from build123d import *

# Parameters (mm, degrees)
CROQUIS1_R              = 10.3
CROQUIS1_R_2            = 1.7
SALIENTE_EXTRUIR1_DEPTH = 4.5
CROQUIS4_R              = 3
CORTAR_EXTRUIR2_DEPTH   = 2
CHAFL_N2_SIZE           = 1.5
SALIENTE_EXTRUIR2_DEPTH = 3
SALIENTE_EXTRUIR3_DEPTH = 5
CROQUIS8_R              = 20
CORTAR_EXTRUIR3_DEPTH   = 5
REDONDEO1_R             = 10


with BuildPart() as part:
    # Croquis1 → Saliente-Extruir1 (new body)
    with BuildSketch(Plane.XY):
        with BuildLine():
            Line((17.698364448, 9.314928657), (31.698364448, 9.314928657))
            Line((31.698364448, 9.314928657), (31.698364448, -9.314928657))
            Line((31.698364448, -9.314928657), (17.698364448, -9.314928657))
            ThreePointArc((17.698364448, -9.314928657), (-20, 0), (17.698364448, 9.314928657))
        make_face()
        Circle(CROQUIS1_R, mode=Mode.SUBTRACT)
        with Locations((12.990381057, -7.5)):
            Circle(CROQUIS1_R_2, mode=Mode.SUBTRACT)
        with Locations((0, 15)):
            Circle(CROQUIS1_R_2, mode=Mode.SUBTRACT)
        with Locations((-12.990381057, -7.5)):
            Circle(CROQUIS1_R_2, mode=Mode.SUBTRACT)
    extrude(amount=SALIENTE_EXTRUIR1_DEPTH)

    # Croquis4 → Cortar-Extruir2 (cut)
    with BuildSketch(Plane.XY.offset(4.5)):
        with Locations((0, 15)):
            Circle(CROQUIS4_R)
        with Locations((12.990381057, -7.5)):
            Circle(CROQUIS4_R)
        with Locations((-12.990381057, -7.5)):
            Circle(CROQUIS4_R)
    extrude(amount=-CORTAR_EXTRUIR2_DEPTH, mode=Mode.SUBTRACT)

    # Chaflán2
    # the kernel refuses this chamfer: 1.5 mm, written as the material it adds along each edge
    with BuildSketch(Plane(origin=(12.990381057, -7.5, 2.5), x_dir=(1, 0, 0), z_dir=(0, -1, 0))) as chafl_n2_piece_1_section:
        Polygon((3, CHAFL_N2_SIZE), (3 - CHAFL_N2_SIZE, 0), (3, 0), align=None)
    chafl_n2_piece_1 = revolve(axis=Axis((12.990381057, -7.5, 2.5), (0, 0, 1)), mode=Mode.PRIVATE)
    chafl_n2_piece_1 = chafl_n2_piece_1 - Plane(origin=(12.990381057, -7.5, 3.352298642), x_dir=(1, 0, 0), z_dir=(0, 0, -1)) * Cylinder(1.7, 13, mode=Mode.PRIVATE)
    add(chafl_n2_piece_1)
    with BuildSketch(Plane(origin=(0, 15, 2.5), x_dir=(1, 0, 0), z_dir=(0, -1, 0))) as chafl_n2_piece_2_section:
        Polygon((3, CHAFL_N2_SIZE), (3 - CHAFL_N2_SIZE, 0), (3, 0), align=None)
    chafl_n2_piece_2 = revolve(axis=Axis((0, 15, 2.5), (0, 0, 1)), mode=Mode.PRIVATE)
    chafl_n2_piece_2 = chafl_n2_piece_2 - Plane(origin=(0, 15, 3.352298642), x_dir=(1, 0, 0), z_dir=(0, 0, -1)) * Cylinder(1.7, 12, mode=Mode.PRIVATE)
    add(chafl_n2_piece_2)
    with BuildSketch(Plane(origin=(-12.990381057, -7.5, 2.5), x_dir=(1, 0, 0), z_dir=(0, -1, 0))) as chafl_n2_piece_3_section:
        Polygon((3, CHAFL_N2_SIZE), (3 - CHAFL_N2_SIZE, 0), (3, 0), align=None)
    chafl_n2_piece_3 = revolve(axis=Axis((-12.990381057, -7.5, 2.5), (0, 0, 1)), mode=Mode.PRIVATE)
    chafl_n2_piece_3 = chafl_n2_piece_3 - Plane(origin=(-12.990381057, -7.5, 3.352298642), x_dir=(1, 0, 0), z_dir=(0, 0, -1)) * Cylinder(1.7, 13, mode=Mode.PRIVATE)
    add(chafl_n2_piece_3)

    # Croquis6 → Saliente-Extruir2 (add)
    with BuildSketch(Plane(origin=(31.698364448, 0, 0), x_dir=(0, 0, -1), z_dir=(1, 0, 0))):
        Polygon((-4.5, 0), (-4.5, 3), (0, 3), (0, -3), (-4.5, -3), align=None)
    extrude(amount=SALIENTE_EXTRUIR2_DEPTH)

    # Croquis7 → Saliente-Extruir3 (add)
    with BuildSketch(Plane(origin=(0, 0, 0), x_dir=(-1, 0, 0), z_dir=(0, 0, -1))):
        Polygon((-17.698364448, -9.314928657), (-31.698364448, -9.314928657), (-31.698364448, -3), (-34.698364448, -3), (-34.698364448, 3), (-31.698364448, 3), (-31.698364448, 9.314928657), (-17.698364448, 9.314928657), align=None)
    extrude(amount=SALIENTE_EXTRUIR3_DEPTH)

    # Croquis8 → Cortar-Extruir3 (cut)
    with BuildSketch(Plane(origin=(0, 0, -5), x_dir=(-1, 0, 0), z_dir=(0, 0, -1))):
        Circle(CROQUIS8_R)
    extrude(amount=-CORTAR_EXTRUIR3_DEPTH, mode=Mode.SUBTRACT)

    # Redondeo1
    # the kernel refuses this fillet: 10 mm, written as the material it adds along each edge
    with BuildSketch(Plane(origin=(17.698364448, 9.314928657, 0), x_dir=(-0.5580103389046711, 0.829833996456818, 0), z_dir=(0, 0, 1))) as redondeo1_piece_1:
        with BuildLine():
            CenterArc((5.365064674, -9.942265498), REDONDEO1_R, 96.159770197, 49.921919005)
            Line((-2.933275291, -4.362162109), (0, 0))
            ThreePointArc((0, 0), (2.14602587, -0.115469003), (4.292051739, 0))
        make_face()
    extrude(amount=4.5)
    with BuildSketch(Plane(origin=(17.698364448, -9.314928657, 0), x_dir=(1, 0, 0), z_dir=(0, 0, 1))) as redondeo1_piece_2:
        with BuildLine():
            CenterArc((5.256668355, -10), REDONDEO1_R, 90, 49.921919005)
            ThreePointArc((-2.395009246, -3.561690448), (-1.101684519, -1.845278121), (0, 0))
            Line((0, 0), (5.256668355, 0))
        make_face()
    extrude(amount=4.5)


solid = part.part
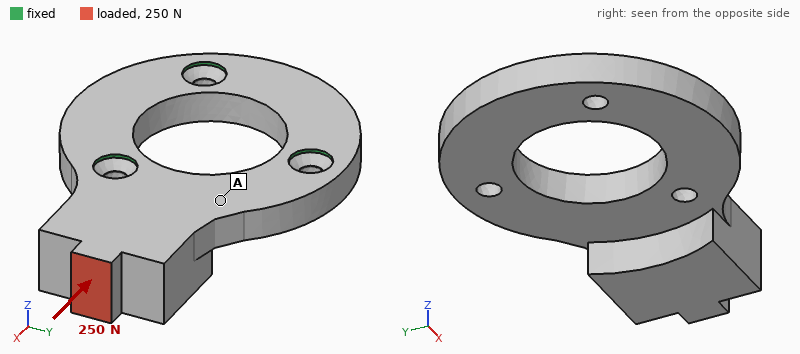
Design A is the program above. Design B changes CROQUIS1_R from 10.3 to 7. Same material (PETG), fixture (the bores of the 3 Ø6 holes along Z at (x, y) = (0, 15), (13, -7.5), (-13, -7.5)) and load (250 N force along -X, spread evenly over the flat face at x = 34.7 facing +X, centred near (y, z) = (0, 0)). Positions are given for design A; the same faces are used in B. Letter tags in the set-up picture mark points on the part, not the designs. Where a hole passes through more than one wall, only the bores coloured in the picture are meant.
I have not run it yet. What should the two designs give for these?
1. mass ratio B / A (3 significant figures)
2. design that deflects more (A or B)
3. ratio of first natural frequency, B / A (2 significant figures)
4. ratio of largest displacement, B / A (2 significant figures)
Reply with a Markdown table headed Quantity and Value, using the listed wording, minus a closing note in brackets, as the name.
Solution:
| Quantity | Value |
|---|---|
| mass ratio B / A | 1.13 |
| design that deflects more | A |
| ratio of first natural frequency, B / A | 1.1 |
| ratio of largest displacement, B / A | 0.86 |
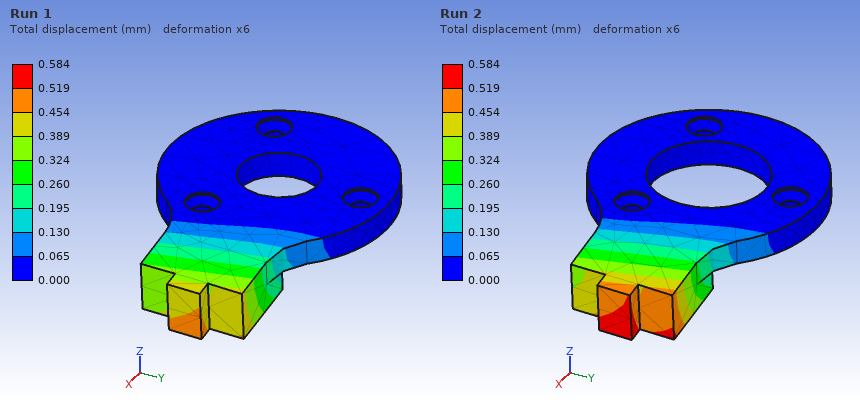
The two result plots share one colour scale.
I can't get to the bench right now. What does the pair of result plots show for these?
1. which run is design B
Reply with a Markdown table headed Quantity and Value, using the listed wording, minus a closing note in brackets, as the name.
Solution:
| Quantity | Value |
|---|---|
| which run is design B | Run 1 |
